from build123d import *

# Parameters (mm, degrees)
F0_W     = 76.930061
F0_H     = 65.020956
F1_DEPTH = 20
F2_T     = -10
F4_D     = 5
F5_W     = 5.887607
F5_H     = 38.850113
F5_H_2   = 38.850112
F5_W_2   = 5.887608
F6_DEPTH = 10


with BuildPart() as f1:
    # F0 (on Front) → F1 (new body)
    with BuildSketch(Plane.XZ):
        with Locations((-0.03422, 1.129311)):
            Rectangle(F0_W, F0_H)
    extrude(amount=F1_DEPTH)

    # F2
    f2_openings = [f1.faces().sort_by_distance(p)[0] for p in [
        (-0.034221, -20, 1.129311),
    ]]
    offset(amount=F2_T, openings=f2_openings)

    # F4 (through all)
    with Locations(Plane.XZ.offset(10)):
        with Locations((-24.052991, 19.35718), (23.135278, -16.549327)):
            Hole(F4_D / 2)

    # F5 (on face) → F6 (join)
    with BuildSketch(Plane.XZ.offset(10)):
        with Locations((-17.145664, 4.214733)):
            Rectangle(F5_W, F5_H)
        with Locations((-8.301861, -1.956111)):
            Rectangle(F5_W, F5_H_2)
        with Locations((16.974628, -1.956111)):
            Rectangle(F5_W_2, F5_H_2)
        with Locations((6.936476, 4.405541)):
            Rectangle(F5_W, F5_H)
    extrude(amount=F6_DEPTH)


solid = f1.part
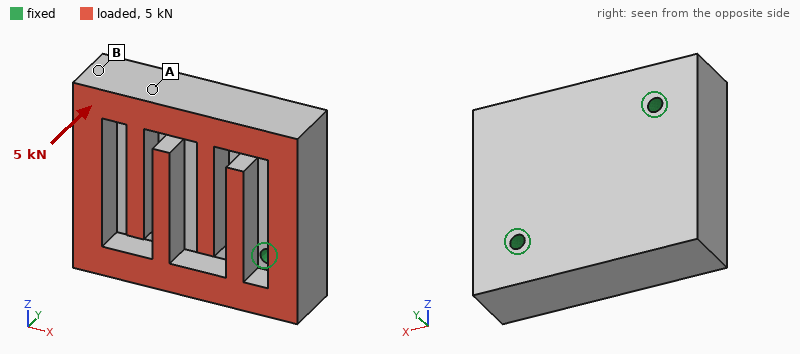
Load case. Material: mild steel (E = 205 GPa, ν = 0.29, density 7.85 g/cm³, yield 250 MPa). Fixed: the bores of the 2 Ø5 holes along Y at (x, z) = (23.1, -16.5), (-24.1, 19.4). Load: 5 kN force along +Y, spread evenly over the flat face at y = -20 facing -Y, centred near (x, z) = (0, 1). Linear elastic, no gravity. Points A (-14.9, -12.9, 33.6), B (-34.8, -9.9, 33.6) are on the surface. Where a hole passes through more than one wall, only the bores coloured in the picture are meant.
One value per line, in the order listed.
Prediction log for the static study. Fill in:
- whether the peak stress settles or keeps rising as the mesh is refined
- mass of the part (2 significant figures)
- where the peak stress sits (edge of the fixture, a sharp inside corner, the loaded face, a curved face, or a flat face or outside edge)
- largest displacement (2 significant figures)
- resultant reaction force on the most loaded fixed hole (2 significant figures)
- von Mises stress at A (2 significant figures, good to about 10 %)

keeps rising
650 g
edge of the fixture
13 µm
2.5 kN
11 MPa
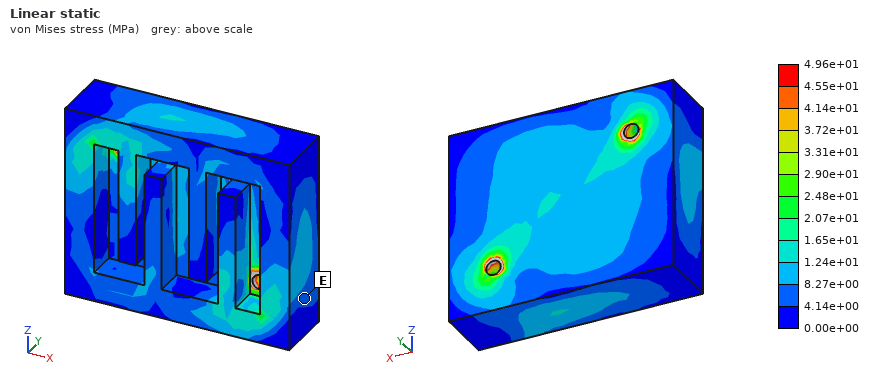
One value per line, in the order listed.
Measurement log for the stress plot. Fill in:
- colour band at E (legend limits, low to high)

4.14e+00 to 8.27e+00 MPa
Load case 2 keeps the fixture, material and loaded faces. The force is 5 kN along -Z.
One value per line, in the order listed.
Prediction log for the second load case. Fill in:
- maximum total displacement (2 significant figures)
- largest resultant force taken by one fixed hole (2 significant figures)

21 µm
2.6 kN
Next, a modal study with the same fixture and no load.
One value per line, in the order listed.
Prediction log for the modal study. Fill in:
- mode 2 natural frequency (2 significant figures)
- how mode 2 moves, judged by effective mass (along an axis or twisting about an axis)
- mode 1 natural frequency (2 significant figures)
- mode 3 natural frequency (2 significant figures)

5300 Hz
along Y
3500 Hz
12 kHz
